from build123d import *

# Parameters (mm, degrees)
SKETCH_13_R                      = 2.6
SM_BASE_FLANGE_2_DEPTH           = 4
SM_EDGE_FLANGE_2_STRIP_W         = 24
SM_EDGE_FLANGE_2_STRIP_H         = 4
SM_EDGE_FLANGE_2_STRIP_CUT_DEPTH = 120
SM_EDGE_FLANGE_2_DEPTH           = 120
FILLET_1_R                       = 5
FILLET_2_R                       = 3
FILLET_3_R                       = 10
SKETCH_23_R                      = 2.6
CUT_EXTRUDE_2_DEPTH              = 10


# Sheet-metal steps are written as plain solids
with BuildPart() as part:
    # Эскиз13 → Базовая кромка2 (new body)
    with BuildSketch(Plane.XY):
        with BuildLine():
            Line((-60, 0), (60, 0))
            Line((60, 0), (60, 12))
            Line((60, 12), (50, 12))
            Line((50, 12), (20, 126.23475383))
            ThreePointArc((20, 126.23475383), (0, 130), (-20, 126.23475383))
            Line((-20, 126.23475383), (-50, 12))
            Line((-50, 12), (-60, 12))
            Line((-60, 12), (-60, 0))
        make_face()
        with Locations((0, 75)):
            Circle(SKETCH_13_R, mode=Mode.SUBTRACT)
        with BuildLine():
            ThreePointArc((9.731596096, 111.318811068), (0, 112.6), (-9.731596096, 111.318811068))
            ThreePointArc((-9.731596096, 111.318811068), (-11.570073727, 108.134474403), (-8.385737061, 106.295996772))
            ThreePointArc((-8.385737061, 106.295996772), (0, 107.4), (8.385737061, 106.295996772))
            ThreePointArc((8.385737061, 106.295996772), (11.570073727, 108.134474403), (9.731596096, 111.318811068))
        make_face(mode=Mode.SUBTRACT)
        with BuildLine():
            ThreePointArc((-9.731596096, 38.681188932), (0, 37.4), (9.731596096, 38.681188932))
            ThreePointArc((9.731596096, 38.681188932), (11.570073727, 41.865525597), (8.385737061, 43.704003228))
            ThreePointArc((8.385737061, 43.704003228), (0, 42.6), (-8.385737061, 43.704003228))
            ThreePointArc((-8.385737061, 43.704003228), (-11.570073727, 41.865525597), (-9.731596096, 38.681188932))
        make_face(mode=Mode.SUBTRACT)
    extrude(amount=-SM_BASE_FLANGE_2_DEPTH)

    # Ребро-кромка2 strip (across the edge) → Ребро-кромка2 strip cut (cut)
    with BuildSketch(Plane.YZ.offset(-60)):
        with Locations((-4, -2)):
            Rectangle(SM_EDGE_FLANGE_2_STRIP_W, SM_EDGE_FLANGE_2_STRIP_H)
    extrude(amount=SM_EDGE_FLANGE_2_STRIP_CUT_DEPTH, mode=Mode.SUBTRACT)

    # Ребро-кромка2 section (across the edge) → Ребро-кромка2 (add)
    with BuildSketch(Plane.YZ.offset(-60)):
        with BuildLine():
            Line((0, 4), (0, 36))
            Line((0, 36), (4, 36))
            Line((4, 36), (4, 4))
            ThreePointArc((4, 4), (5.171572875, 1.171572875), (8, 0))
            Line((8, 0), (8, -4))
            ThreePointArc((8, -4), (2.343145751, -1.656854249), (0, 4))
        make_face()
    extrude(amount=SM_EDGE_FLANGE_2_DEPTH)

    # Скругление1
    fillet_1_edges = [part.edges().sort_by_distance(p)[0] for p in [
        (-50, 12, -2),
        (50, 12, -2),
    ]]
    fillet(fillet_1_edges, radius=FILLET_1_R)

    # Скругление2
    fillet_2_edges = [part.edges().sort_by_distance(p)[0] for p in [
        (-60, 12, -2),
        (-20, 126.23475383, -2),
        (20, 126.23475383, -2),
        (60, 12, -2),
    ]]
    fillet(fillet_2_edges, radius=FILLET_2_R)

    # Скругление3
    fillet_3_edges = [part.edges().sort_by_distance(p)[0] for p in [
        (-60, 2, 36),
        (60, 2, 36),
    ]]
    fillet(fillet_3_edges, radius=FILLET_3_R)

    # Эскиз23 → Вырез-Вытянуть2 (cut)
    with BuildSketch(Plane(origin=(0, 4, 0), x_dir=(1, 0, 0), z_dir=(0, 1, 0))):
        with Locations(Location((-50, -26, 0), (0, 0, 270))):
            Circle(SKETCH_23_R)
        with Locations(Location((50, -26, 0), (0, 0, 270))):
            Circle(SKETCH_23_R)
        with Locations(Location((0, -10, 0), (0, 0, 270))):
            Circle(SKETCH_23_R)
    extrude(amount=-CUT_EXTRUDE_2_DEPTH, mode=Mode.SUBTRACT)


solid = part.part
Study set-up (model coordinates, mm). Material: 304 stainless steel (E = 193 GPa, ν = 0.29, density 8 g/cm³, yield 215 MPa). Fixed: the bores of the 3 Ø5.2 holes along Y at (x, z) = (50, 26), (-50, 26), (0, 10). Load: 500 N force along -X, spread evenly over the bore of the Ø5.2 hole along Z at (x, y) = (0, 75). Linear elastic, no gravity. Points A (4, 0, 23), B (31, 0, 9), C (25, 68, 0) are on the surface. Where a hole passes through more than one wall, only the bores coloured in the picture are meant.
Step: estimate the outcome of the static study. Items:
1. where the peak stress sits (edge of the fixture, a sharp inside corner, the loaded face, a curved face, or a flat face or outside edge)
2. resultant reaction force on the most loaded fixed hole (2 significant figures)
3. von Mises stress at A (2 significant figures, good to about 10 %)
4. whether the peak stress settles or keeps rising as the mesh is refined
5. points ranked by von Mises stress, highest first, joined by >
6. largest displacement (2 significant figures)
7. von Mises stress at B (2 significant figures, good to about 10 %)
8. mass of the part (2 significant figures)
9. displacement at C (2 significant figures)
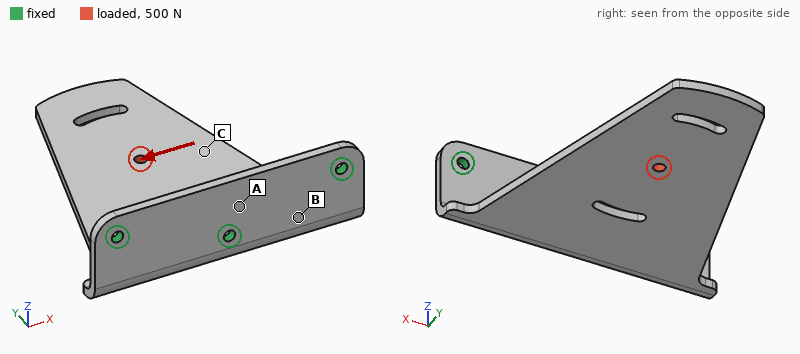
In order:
edge of the fixture
350 N
12 MPa
keeps rising
B > A > C
0.13 mm
23 MPa
420 g
0.077 mm
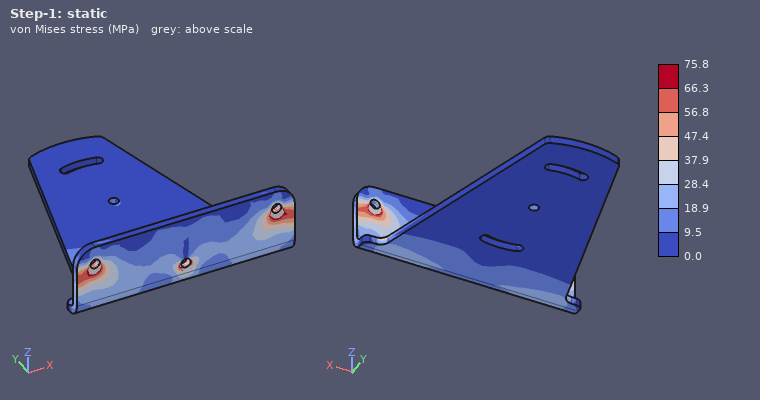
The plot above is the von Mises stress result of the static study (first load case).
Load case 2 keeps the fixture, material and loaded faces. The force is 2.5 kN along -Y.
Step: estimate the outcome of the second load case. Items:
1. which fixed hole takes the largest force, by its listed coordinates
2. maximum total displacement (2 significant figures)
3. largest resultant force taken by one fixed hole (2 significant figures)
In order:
(0, 10)
0.39 mm
2.5 kN
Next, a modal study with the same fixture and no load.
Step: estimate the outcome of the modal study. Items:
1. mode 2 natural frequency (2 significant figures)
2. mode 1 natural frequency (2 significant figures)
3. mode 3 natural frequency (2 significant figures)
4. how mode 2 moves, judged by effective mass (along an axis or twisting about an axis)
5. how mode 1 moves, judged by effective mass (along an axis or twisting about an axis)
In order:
780 Hz
230 Hz
1100 Hz
along X
along Z
